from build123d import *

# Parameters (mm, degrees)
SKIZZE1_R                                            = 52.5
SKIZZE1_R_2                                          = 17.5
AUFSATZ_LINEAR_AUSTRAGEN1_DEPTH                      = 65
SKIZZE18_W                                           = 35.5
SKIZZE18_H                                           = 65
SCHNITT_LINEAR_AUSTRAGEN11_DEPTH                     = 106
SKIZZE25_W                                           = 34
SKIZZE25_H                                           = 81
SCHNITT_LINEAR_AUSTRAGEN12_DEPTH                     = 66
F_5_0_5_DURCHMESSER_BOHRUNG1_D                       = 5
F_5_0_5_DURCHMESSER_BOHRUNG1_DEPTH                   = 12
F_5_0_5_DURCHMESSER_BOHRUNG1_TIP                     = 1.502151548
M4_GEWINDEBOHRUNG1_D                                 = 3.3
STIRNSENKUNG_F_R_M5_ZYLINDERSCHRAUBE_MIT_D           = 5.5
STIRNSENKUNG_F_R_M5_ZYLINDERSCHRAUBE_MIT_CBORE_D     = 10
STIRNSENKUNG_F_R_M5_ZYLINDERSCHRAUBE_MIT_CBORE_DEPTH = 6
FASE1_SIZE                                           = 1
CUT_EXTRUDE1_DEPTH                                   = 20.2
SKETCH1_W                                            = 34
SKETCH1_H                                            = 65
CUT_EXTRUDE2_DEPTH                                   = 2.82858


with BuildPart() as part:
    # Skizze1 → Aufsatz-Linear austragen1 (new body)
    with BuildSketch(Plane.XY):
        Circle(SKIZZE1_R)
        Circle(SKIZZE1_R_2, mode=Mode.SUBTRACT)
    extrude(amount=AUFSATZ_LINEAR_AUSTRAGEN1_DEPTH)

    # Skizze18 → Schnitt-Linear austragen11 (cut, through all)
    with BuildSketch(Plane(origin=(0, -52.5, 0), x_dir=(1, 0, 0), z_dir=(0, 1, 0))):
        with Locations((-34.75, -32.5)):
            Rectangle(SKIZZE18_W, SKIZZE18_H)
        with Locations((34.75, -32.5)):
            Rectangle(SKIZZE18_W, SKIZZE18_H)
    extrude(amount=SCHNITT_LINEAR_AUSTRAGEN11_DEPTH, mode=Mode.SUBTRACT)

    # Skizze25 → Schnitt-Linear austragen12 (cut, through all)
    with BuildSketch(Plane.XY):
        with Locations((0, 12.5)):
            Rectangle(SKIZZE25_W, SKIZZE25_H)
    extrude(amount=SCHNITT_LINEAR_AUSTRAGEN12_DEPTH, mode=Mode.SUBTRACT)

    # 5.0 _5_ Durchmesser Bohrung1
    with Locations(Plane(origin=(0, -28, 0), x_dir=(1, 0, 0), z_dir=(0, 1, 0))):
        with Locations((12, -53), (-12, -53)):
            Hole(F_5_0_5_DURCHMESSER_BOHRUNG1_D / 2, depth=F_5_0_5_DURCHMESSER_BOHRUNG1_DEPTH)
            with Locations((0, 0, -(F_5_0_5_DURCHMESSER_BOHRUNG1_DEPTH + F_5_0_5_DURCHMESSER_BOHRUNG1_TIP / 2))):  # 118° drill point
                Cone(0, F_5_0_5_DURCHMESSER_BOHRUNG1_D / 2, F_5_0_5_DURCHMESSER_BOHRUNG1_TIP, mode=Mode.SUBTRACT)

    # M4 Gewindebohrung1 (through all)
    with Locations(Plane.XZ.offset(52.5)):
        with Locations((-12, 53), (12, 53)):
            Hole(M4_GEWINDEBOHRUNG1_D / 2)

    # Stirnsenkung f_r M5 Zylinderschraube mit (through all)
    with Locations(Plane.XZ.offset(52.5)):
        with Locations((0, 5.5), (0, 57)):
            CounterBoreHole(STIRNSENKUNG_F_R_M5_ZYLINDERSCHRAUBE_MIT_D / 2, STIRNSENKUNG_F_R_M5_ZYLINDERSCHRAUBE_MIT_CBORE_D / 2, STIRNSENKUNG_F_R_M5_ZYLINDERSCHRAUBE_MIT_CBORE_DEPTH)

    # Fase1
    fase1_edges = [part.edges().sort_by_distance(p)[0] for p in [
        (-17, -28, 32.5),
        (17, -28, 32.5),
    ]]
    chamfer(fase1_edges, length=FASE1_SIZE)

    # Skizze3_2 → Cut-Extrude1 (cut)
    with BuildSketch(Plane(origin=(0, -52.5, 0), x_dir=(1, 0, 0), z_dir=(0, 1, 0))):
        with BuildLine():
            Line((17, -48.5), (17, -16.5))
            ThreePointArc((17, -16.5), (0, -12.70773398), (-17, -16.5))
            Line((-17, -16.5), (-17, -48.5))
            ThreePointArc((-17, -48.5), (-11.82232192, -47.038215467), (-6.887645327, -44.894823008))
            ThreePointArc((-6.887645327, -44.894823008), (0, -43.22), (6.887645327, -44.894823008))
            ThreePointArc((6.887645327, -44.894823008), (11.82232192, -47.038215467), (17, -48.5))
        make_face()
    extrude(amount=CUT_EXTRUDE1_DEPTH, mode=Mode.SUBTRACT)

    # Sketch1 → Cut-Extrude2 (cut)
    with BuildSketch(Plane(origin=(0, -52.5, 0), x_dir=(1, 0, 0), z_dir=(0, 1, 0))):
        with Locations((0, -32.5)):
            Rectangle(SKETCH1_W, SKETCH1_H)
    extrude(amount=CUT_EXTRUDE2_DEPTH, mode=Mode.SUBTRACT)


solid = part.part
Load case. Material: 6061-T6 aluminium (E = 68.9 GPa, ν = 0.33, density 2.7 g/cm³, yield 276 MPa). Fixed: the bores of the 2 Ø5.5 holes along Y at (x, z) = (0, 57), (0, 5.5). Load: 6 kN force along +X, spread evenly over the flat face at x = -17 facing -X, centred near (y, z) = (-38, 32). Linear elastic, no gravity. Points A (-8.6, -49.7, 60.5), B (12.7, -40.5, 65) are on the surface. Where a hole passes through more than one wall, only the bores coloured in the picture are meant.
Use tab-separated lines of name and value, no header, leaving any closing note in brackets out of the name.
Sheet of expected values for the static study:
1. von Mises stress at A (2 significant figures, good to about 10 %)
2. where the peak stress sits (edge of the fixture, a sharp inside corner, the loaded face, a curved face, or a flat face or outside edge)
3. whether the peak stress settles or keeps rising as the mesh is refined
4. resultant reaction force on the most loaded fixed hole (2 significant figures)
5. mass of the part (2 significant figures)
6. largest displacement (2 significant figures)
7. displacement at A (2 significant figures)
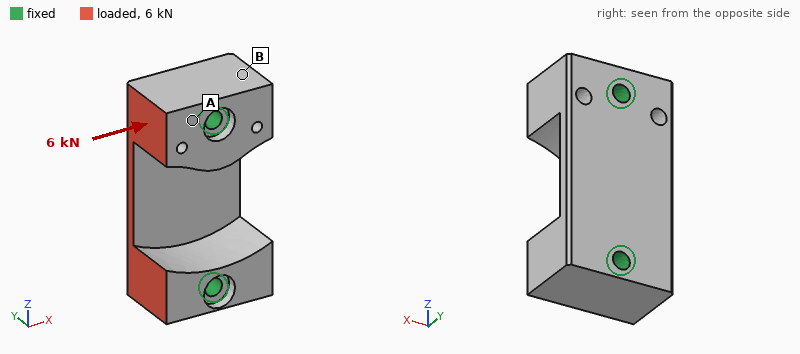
von Mises stress at A	5.8 MPa
where the peak stress sits	edge of the fixture
whether the peak stress settles or keeps rising as the mesh is refined	keeps rising
resultant reaction force on the most loaded fixed hole	3.1 kN
mass of the part	73 g
largest displacement	8.3 µm
displacement at A	1.8 µm
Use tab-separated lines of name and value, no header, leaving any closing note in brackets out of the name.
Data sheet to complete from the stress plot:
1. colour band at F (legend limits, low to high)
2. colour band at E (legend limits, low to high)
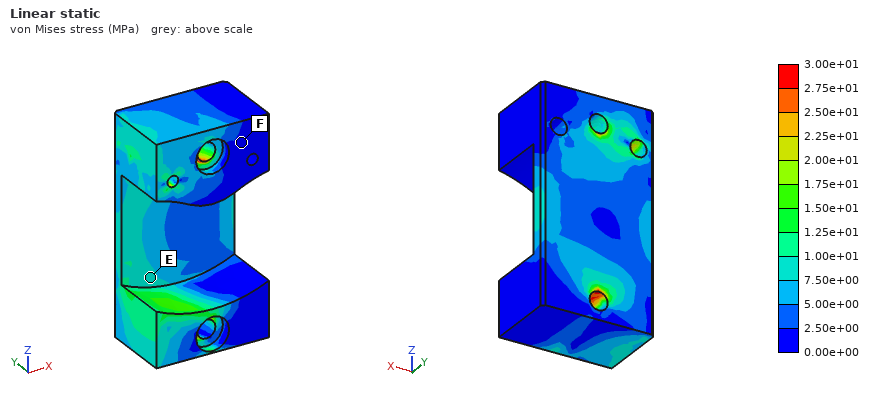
colour band at F	0.00e+00 to 2.50e+00 MPa
colour band at E	7.50e+00 to 1.00e+01 MPa
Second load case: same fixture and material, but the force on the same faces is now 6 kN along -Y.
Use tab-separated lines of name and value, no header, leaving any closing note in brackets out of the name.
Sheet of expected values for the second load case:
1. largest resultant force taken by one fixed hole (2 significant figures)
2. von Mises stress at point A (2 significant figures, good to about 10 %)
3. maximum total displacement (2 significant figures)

largest resultant force taken by one fixed hole	3.1 kN
von Mises stress at point A	16 MPa
maximum total displacement	53 µm
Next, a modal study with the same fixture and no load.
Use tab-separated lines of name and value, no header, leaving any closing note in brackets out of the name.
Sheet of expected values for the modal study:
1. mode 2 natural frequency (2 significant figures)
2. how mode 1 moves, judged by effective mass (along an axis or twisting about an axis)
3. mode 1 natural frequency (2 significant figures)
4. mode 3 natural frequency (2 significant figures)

mode 2 natural frequency	17 kHz
how mode 1 moves, judged by effective mass	along Y
mode 1 natural frequency	15 kHz
mode 3 natural frequency	20 kHz
